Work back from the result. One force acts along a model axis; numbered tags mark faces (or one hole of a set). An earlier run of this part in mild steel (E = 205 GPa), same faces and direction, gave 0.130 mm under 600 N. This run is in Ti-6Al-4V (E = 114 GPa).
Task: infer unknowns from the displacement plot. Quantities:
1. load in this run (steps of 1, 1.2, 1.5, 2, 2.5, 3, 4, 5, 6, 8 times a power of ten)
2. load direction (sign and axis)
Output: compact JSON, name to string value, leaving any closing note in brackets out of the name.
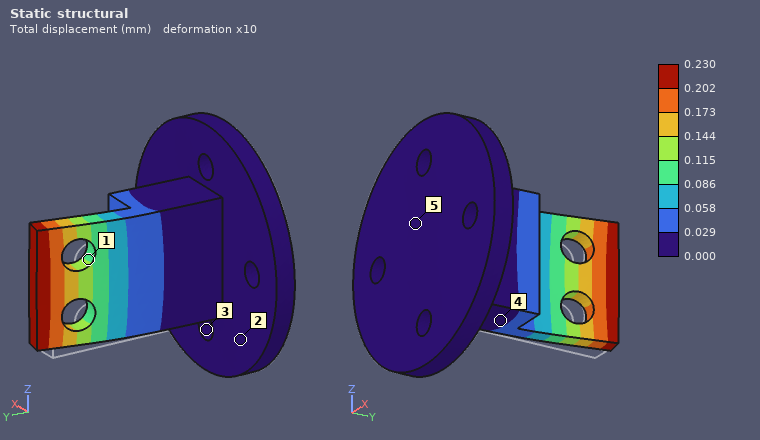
{"load in this run": "600 N", "load direction": "+X"}
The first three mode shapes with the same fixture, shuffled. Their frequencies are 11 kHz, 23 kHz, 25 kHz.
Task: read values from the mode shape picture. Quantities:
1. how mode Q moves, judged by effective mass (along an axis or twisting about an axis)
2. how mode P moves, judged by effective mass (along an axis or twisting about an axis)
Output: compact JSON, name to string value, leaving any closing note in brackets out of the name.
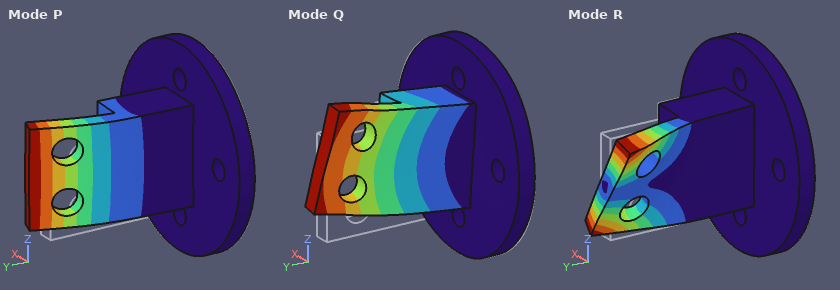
{"how mode Q moves, judged by effective mass": "along Z", "how mode P moves, judged by effective mass": "along X"}
